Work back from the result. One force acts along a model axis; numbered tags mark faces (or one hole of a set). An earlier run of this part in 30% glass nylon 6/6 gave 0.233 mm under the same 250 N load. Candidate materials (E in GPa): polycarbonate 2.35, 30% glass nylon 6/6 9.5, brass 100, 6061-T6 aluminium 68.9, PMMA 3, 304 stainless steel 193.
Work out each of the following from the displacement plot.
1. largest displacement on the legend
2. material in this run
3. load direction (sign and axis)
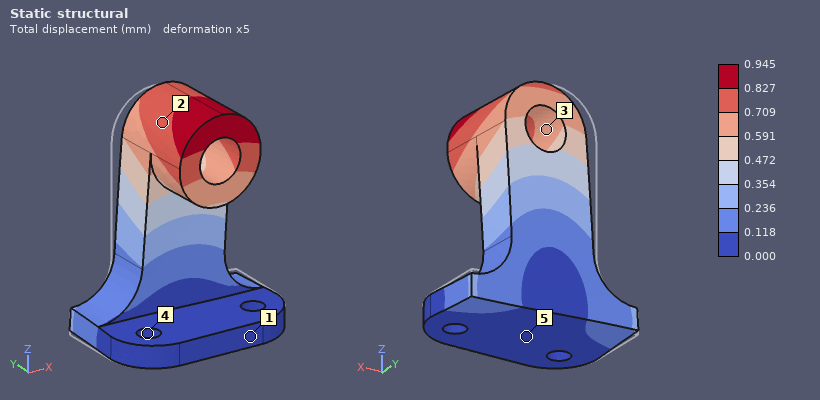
0.945 mm
polycarbonate
+X
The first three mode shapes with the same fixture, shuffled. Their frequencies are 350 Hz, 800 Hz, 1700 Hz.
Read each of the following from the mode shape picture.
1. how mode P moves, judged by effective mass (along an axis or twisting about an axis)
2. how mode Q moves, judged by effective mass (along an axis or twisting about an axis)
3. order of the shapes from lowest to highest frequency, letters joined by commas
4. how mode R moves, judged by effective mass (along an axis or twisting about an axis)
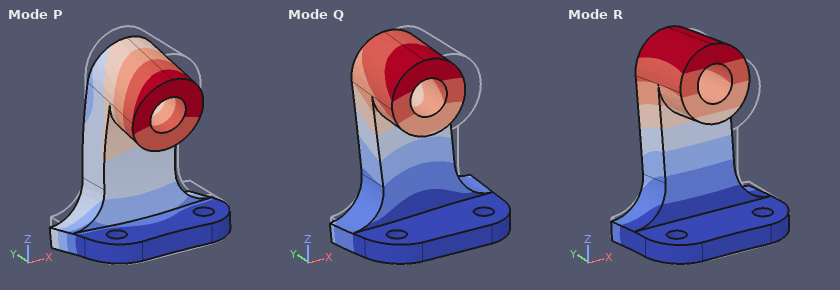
along Z
along X
R, Q, P
along Y
